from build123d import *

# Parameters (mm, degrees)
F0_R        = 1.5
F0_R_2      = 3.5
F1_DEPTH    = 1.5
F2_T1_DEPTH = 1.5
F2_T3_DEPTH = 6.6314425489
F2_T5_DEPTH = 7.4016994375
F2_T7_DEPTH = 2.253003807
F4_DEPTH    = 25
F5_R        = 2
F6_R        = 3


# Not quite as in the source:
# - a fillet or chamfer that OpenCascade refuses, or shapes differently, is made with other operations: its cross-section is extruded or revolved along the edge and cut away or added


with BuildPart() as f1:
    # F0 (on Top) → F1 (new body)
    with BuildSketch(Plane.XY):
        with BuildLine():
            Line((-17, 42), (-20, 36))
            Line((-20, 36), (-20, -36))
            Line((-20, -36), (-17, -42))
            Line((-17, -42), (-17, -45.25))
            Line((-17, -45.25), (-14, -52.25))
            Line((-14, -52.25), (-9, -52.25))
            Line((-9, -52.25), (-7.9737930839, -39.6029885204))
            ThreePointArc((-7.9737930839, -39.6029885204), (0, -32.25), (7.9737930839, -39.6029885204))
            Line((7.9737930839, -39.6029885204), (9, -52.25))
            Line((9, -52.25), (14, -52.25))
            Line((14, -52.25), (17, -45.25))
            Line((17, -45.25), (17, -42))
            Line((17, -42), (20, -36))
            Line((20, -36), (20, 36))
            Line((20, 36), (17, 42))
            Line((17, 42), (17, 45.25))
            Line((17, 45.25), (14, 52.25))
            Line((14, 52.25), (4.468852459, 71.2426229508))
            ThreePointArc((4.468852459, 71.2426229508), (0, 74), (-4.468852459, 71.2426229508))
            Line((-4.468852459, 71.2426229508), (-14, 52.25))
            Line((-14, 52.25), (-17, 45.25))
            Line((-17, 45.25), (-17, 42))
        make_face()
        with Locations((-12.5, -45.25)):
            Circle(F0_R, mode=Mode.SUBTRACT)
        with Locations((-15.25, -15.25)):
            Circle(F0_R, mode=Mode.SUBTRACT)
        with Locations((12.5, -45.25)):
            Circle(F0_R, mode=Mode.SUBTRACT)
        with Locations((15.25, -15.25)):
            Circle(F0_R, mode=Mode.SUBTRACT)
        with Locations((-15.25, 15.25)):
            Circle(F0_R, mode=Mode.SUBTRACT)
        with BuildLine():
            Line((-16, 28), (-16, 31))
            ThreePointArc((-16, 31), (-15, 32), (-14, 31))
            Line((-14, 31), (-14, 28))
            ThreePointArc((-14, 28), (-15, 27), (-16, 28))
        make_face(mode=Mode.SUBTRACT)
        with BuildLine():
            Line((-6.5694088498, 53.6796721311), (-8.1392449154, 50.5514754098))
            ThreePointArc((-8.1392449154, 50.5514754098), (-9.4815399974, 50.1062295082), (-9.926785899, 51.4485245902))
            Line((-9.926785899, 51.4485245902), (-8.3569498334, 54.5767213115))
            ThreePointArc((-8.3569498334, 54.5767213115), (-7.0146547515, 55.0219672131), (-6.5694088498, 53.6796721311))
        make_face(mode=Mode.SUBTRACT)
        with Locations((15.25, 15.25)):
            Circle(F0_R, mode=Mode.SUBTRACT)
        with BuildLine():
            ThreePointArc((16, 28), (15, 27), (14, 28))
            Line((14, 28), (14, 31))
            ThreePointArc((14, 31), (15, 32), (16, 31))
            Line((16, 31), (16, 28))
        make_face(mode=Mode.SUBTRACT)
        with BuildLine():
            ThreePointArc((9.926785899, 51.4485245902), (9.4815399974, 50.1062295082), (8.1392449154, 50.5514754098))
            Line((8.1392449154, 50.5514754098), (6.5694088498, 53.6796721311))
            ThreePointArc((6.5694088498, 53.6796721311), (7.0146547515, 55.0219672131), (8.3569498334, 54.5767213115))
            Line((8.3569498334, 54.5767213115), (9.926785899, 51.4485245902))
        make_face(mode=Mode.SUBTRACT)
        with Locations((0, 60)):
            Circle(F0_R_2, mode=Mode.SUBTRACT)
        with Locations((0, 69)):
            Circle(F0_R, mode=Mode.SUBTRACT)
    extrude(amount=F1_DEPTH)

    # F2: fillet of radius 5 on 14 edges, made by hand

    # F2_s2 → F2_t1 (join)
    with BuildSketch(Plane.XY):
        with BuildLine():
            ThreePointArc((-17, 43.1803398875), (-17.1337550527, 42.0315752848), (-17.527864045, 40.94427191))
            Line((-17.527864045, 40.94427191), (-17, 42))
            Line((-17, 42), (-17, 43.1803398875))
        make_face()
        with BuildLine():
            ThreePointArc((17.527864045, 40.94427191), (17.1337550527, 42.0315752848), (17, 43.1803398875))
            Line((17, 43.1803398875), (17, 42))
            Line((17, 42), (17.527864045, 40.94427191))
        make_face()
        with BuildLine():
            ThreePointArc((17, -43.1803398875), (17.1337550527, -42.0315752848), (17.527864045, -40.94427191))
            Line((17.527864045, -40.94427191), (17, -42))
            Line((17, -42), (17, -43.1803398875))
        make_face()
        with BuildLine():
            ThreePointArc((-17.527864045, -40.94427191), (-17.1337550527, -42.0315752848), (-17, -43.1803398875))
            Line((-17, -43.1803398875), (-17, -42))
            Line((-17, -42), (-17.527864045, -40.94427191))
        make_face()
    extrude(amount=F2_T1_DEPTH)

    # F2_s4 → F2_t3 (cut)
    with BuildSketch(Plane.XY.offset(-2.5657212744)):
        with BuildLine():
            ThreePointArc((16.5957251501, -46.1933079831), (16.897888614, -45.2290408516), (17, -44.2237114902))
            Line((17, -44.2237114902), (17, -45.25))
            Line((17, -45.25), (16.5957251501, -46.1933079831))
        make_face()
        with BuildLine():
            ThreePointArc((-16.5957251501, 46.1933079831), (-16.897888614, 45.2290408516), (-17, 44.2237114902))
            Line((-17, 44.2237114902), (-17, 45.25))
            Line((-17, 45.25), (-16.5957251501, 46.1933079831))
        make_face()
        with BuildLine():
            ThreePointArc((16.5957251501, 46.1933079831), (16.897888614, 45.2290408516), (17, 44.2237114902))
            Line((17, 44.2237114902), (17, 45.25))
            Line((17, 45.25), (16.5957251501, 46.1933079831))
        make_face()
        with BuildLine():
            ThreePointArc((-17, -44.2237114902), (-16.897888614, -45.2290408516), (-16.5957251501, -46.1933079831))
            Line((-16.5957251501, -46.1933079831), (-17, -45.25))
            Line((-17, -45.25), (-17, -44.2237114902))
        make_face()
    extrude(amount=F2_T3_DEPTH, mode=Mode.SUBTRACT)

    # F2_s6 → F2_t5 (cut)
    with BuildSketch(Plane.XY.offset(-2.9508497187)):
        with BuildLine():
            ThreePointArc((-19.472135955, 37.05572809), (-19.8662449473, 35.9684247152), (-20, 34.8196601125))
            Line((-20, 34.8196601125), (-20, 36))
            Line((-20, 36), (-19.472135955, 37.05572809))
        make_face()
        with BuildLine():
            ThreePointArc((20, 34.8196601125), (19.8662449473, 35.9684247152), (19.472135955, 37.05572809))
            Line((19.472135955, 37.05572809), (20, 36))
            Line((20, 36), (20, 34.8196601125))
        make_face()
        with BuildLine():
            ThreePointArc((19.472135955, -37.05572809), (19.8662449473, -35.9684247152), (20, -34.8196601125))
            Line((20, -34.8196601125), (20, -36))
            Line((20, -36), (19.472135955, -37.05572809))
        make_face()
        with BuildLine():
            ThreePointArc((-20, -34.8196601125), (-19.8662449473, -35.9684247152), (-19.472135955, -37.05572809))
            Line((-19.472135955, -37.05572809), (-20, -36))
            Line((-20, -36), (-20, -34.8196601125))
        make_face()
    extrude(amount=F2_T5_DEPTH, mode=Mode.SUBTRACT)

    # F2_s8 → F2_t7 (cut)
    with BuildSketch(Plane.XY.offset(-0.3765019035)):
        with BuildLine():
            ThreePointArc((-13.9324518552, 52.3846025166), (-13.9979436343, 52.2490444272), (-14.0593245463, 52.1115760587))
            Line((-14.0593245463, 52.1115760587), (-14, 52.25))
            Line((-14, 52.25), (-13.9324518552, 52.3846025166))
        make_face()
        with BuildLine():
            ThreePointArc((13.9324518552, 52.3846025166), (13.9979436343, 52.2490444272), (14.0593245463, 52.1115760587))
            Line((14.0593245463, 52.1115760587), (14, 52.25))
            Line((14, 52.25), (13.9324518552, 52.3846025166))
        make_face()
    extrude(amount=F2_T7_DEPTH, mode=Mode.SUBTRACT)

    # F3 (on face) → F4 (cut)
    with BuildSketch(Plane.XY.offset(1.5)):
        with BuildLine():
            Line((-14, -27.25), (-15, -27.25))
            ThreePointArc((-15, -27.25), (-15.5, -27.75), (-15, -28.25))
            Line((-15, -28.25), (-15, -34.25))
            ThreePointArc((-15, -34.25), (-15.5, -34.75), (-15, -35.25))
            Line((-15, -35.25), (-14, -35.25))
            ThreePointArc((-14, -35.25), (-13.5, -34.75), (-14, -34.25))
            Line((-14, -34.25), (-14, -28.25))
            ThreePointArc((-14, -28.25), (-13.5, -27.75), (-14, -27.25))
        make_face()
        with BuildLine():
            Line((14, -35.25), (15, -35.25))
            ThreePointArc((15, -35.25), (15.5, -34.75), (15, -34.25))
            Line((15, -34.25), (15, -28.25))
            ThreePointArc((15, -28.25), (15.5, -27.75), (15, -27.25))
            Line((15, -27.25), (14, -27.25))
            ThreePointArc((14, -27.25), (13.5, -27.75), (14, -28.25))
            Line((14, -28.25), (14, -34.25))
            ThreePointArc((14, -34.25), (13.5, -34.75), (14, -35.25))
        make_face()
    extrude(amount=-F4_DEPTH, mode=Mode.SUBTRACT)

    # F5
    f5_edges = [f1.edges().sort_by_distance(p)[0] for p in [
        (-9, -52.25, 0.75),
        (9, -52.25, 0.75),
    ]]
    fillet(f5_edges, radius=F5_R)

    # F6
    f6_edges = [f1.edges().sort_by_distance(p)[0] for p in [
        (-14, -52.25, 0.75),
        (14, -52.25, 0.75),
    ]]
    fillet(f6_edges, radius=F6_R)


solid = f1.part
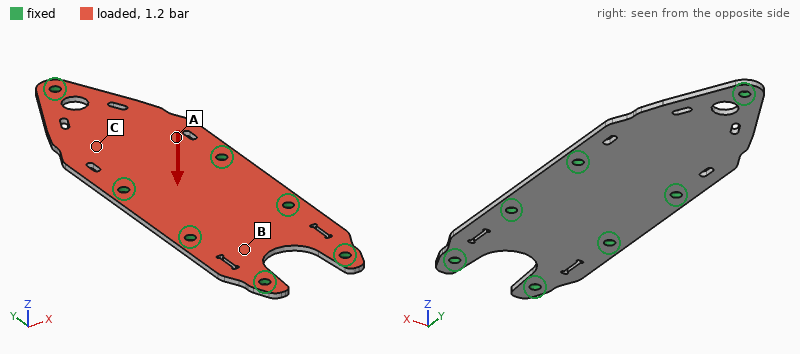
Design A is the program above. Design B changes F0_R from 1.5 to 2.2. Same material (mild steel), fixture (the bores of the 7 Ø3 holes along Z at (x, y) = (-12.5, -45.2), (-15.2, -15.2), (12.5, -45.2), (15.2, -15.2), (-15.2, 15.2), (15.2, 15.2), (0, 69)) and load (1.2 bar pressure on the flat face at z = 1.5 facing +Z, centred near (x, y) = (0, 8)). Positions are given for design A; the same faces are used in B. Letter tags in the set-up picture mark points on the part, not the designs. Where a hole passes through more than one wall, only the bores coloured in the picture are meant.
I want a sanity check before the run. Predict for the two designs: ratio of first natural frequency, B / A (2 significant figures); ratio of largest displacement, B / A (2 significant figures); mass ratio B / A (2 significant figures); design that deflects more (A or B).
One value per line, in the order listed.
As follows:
1.1
0.90
0.99
A
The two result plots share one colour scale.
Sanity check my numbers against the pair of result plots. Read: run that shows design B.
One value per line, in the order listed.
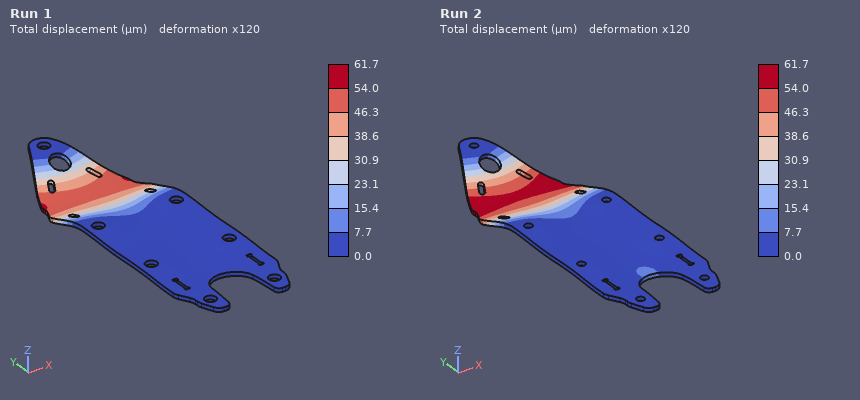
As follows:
Run 1
